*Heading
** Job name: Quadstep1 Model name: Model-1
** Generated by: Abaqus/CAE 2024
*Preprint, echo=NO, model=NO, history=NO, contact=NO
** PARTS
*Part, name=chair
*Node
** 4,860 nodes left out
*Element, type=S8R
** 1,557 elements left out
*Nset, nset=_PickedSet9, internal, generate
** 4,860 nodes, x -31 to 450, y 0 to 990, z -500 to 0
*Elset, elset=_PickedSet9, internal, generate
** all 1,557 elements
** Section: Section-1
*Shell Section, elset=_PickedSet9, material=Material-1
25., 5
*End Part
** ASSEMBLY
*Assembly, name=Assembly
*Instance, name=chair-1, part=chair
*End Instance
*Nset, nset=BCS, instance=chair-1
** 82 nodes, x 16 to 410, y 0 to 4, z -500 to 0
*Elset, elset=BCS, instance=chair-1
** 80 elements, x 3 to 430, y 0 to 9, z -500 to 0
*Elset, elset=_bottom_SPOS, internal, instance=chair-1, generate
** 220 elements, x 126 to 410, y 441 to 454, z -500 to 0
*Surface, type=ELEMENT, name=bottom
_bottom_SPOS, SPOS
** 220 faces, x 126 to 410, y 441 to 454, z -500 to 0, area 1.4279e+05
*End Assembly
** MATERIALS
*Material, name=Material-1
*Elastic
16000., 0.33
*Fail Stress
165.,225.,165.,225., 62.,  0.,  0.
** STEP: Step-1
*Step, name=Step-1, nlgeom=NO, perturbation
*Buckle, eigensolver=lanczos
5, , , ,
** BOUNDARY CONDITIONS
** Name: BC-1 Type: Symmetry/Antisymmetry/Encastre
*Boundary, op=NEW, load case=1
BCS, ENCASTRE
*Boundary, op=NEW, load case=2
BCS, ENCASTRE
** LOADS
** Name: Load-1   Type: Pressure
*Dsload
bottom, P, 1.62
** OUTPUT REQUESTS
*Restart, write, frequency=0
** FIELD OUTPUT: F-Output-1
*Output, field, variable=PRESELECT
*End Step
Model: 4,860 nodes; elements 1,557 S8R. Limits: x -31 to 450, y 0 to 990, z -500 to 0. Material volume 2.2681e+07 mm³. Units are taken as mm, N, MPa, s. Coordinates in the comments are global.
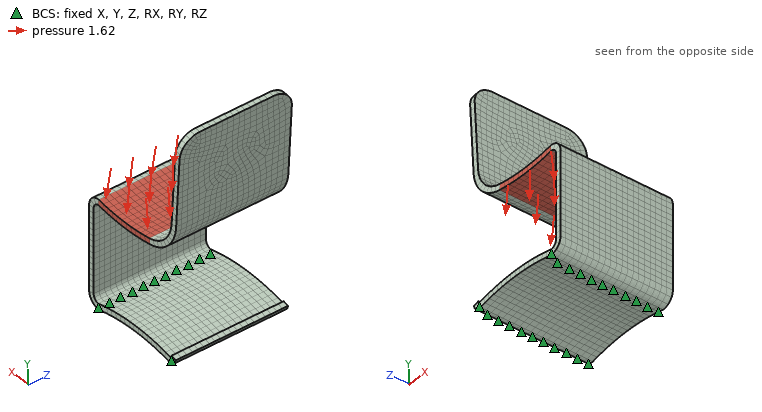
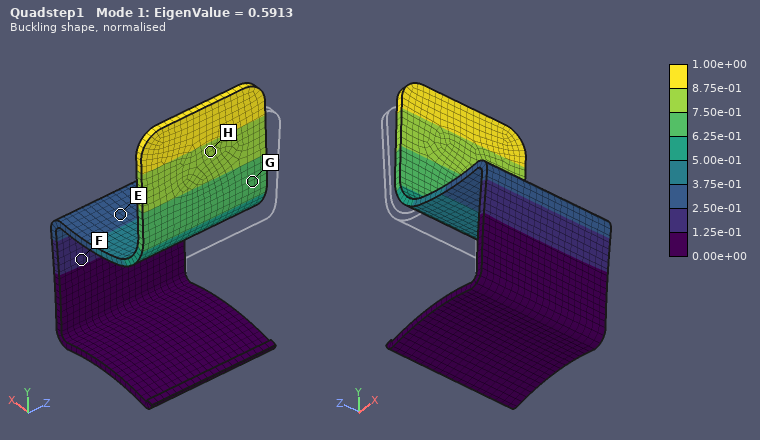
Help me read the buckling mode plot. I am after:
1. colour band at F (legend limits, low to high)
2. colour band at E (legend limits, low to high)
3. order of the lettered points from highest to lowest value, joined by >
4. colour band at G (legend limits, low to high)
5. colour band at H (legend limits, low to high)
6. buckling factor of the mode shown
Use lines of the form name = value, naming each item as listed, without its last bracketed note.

colour band at F = 1.25e-01 to 2.50e-01
colour band at E = 2.50e-01 to 3.75e-01
order of the lettered points from highest to lowest value, joined by > = H > G > E > F
colour band at G = 6.25e-01 to 7.50e-01
colour band at H = 7.50e-01 to 8.75e-01
buckling factor of the mode shown = 0.5913
